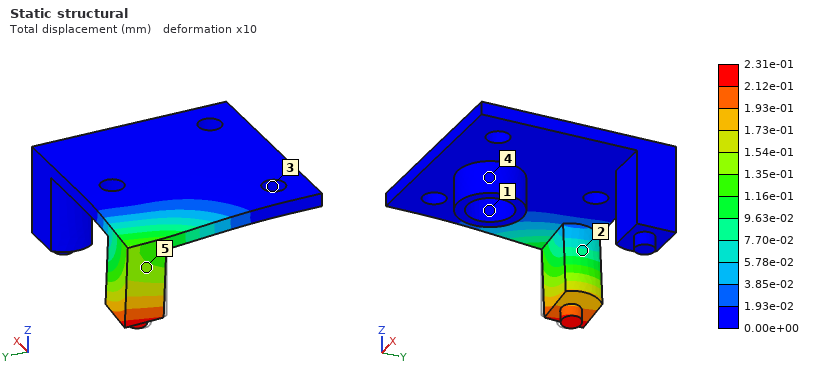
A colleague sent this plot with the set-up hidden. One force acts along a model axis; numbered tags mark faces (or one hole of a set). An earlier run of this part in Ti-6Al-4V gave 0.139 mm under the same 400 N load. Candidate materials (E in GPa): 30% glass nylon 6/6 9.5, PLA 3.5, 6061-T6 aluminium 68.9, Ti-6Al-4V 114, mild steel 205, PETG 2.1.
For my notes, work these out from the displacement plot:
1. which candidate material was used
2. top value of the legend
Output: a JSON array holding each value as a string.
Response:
["6061-T6 aluminium", "2.31e-01 mm"]
